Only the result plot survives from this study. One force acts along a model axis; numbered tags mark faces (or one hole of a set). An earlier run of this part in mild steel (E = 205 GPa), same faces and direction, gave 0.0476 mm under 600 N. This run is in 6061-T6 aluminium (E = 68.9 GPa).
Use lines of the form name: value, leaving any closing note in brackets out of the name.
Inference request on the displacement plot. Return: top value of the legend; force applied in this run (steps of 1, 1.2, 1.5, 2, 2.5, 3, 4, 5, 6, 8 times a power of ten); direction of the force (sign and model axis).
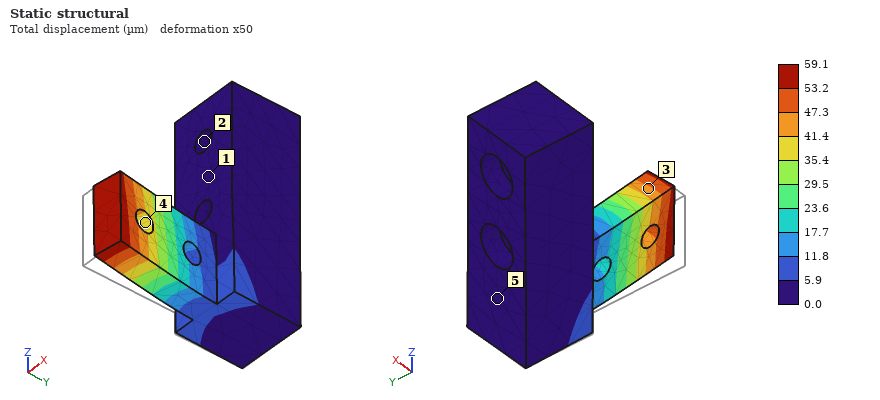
top value of the legend: 59.1 µm
force applied in this run: 250 N
direction of the force: +X
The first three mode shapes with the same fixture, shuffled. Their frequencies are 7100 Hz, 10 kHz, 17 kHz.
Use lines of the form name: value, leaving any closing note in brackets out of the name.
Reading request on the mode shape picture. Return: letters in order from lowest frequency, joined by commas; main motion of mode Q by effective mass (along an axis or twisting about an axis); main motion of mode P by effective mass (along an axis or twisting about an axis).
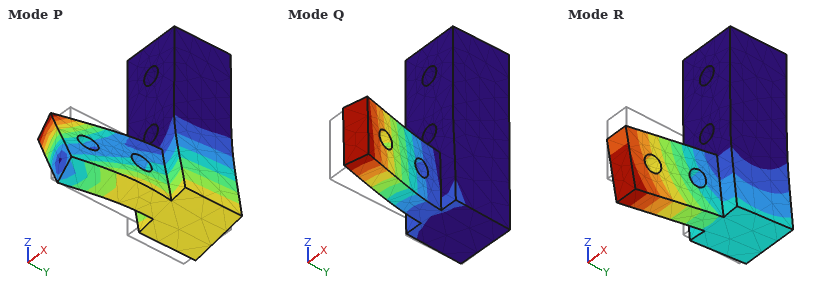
letters in order from lowest frequency, joined by commas: Q, R, P
main motion of mode Q by effective mass: along X
main motion of mode P by effective mass: along X
